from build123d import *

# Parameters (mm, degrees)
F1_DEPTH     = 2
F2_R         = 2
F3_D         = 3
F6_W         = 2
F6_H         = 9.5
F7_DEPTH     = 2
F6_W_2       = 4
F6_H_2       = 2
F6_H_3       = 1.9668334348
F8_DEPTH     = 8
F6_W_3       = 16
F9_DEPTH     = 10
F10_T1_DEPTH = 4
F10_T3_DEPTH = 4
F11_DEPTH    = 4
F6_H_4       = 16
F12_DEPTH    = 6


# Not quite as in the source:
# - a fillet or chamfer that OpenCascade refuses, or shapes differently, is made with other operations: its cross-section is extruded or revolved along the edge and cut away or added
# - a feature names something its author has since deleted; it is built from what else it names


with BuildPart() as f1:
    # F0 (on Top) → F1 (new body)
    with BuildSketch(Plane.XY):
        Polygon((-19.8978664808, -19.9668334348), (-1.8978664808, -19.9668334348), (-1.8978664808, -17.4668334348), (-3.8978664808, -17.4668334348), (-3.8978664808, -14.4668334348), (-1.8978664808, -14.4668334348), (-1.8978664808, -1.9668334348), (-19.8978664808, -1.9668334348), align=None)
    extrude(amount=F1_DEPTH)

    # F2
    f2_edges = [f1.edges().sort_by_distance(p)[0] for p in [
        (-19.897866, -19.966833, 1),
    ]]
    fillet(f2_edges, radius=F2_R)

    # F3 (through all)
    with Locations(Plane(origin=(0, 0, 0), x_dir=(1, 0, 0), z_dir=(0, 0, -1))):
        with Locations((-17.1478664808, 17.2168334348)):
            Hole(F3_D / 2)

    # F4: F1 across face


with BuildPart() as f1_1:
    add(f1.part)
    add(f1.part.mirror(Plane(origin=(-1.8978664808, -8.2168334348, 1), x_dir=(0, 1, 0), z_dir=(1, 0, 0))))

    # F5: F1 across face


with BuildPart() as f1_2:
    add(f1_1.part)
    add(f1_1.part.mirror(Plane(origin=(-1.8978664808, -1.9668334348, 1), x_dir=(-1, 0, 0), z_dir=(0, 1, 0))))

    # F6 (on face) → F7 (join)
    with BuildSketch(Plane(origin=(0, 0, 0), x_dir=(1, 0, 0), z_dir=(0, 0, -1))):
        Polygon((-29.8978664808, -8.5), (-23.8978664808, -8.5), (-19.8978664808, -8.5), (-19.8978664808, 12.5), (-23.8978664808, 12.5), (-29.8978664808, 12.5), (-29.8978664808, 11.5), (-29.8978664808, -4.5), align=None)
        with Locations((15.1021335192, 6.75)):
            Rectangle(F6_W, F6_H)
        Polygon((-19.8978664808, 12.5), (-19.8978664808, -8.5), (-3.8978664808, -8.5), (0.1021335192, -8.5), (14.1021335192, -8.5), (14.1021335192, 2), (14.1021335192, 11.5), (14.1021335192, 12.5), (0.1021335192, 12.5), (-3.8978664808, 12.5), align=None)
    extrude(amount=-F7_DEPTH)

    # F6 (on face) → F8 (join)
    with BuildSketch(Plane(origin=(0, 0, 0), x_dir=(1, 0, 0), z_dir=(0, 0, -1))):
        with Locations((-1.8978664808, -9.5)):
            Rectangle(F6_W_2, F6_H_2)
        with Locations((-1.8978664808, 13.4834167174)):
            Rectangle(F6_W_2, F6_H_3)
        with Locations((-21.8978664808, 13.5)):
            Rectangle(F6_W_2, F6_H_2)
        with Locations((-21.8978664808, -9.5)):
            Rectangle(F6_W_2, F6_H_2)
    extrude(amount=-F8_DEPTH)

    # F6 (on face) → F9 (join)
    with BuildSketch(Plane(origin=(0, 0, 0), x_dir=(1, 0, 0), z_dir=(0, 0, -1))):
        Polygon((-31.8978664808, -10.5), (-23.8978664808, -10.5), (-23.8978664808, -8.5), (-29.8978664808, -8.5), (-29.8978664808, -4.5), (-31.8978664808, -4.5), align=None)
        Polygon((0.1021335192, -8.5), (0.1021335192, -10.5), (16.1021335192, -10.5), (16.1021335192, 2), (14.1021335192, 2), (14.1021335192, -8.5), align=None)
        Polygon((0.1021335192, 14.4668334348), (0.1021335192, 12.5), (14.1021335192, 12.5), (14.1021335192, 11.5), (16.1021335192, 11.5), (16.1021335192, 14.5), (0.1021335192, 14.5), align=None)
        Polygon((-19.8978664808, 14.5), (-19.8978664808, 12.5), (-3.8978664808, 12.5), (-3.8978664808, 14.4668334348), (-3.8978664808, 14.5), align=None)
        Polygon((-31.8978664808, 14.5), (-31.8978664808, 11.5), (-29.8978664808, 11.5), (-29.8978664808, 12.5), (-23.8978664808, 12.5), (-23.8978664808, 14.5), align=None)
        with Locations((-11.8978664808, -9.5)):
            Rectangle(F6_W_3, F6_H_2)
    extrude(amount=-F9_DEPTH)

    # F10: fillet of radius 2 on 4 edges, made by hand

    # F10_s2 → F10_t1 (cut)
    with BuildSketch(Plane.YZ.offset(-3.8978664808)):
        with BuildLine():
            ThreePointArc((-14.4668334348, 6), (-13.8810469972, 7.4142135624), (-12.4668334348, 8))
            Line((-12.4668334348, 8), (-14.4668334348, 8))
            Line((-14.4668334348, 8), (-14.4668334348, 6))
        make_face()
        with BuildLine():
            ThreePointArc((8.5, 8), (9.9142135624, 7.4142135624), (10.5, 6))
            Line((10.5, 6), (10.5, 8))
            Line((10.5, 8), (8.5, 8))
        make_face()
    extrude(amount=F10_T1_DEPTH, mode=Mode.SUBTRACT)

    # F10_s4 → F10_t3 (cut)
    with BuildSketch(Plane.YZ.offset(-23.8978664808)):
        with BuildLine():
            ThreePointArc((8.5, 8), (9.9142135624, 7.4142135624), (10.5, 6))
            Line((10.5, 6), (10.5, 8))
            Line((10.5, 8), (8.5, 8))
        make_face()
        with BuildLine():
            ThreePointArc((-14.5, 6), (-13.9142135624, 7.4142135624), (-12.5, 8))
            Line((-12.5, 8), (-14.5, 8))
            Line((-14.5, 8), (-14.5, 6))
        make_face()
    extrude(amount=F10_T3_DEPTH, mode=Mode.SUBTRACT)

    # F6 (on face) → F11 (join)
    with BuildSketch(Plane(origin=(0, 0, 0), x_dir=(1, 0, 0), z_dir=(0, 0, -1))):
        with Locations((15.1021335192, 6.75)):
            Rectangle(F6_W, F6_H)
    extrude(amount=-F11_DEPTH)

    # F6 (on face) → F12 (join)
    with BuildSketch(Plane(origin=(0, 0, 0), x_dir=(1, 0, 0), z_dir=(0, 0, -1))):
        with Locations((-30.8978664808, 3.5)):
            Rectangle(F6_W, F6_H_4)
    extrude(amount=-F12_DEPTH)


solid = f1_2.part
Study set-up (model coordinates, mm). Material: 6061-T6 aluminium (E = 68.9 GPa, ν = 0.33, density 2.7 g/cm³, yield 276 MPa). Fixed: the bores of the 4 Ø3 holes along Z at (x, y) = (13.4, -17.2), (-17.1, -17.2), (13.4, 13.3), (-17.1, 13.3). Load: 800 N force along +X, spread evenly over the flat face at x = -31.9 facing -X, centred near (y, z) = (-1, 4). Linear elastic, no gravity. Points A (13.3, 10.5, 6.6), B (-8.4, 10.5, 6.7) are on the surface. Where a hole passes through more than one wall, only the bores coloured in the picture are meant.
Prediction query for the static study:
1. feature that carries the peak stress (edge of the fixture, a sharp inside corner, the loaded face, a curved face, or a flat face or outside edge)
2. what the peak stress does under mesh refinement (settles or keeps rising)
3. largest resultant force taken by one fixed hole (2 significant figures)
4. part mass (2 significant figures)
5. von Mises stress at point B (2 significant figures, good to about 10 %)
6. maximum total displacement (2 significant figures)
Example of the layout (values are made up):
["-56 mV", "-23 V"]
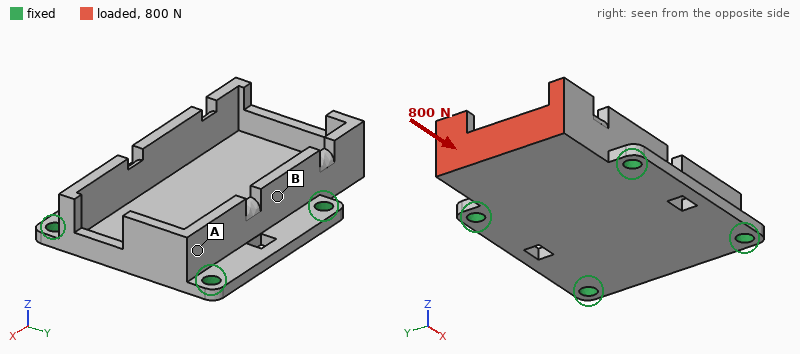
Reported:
["edge of the fixture", "keeps rising", "260 N", "13 g", "14 MPa", "37 µm"]
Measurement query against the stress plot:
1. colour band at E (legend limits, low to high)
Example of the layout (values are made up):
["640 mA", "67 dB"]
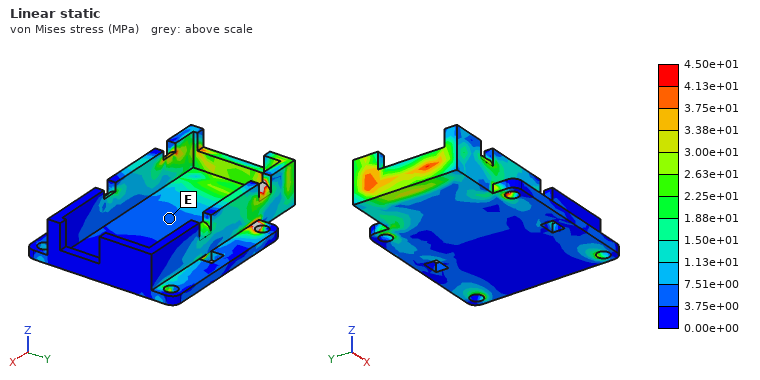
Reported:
["3.75e+00 to 7.51e+00 MPa"]
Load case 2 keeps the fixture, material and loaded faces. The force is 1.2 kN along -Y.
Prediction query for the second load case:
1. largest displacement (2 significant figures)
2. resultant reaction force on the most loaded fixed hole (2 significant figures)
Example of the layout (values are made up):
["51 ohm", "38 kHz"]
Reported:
["78 µm", "860 N"]
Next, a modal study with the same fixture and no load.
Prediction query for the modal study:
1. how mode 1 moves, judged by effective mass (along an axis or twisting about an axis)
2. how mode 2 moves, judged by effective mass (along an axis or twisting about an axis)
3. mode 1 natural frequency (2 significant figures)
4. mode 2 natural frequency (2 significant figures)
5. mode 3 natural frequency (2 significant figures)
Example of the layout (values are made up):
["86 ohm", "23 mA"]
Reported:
["along Z", "along Z", "8400 Hz", "9700 Hz", "13 kHz"]
